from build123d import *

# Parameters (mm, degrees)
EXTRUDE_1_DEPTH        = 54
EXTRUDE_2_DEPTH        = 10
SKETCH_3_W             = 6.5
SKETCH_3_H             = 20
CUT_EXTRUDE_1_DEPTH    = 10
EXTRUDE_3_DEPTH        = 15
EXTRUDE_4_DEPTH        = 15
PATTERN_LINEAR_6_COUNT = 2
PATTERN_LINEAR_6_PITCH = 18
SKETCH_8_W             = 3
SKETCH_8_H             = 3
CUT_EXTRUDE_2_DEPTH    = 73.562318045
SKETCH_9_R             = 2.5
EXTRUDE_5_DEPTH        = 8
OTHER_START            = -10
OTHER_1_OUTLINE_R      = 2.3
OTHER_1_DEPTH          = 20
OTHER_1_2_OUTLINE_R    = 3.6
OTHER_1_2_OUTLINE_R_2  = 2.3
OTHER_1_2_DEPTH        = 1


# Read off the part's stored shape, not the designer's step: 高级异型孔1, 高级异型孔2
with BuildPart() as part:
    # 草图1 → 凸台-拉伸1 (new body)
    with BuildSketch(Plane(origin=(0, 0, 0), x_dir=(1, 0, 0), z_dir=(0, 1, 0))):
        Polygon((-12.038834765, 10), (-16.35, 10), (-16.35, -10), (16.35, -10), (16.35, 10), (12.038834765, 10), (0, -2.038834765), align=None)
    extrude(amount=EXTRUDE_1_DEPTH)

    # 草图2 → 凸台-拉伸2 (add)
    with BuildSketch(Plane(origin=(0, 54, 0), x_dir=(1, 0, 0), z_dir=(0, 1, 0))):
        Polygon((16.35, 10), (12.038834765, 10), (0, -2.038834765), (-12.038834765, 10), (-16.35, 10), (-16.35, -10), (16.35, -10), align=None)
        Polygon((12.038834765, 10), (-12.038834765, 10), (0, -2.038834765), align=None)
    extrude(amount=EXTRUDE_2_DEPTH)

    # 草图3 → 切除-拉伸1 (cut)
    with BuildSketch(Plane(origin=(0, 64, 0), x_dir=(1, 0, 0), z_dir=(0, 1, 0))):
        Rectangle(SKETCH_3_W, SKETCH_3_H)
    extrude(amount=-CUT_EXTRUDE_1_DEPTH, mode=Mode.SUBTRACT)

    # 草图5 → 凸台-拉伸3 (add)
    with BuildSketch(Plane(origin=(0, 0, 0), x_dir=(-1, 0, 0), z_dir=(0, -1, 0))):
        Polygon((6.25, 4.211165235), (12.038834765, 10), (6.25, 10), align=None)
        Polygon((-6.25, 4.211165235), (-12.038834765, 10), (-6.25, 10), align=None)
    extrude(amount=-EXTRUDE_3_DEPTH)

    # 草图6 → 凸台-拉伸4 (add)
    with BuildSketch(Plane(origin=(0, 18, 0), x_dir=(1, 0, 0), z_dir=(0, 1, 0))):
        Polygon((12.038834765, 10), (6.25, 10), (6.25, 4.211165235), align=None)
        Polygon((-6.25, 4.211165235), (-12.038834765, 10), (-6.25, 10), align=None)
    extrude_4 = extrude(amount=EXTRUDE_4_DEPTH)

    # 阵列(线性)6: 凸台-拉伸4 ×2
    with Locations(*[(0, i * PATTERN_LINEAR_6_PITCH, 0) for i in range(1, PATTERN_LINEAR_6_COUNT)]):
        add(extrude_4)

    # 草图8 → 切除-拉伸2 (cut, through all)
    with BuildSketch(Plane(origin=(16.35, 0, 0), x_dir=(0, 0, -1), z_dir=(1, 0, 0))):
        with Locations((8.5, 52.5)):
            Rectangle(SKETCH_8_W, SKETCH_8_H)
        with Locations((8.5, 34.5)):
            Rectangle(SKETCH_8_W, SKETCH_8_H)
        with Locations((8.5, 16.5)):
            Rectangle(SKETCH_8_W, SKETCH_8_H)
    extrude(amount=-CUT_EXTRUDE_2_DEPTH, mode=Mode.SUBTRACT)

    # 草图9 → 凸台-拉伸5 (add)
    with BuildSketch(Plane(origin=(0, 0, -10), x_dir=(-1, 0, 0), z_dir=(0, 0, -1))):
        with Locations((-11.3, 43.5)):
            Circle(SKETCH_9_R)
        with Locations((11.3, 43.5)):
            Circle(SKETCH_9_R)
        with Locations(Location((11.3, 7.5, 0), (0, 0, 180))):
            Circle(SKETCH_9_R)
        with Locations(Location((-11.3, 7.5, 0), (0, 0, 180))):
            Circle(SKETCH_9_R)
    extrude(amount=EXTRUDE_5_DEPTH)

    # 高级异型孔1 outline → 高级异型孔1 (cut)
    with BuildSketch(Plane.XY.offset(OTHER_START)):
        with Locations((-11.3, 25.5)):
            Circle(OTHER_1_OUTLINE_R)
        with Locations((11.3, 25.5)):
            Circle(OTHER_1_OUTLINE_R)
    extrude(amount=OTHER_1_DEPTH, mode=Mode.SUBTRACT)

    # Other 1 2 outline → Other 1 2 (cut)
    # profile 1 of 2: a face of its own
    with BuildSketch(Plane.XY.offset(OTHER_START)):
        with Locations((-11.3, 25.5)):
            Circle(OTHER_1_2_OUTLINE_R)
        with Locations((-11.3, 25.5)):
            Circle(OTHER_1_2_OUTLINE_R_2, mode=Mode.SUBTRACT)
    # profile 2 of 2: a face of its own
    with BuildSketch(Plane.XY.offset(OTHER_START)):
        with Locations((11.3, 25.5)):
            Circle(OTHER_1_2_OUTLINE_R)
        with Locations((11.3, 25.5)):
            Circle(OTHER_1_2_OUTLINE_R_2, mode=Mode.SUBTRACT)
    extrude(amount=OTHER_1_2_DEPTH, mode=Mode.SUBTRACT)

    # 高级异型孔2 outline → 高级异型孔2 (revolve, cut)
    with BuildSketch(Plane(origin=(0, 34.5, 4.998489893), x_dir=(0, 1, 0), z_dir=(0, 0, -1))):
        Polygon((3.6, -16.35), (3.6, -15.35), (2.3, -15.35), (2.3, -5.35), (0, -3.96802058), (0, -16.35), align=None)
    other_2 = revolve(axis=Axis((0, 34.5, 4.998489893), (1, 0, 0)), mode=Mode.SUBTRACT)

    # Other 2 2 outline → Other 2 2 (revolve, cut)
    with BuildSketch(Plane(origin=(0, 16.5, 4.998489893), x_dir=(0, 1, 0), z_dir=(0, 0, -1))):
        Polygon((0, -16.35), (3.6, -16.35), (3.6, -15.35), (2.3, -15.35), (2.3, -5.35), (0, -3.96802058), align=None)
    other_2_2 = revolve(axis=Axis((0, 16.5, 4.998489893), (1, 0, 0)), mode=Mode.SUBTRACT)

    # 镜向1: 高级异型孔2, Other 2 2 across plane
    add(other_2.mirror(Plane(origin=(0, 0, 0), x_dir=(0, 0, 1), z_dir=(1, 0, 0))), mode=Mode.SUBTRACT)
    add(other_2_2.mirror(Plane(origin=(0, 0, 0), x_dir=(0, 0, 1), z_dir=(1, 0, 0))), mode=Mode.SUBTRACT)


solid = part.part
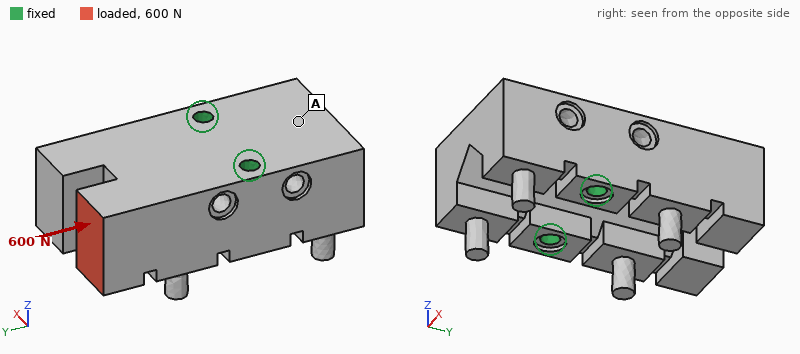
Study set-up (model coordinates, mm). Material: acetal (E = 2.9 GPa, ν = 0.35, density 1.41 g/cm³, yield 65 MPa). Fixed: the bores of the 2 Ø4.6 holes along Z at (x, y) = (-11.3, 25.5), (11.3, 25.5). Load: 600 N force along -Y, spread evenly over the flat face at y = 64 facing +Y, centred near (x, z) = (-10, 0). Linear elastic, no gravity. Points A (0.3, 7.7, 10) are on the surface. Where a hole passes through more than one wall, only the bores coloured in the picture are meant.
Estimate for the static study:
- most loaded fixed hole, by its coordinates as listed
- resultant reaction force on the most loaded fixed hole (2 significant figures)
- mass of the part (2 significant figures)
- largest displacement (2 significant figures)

(-11.3, 25.5)
550 N
47 g
69 µm
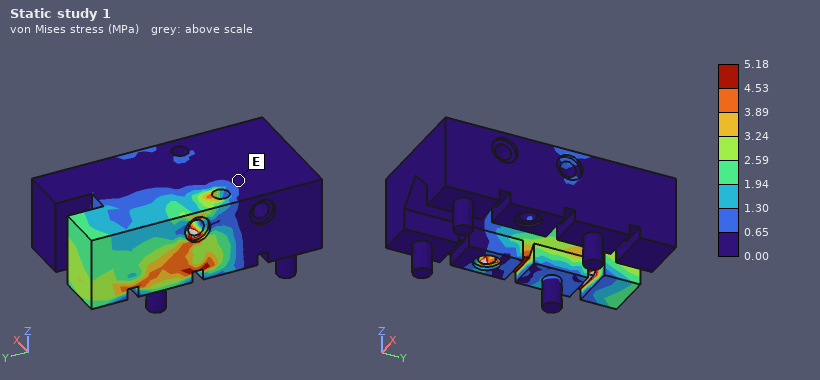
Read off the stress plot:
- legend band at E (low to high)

0.00 to 0.65 MPa
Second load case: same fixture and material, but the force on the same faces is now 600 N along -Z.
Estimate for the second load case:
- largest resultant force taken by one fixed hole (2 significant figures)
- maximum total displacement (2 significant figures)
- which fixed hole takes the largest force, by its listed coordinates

490 N
0.68 mm
(-11.3, 25.5)
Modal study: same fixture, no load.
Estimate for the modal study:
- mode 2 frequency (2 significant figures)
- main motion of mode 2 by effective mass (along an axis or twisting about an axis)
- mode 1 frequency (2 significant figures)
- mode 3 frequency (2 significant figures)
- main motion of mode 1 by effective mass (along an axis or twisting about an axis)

2500 Hz
along X
2200 Hz
3800 Hz
along Z
